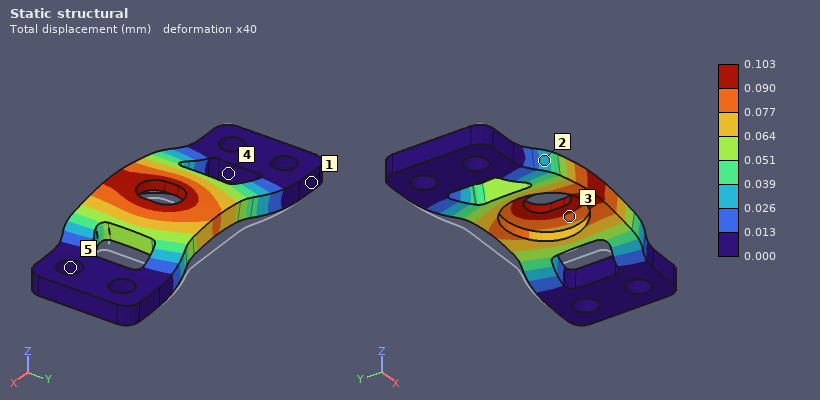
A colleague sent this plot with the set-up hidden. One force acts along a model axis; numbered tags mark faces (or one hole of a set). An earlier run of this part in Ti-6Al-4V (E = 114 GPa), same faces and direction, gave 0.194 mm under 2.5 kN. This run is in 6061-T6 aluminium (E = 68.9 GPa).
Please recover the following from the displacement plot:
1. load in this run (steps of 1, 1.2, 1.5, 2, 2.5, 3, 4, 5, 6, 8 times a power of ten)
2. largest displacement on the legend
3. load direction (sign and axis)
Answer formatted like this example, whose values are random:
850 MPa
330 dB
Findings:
800 N
0.103 mm
+Z
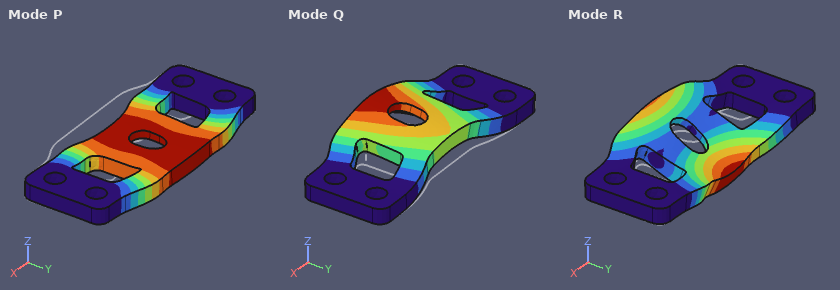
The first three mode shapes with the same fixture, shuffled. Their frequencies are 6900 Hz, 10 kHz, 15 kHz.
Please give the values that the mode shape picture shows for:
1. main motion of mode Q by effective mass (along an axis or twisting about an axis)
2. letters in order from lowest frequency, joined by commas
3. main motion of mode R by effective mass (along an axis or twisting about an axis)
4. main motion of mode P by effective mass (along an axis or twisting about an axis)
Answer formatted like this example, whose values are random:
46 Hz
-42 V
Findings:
along Z
Q, R, P
twisting about X
along Y
